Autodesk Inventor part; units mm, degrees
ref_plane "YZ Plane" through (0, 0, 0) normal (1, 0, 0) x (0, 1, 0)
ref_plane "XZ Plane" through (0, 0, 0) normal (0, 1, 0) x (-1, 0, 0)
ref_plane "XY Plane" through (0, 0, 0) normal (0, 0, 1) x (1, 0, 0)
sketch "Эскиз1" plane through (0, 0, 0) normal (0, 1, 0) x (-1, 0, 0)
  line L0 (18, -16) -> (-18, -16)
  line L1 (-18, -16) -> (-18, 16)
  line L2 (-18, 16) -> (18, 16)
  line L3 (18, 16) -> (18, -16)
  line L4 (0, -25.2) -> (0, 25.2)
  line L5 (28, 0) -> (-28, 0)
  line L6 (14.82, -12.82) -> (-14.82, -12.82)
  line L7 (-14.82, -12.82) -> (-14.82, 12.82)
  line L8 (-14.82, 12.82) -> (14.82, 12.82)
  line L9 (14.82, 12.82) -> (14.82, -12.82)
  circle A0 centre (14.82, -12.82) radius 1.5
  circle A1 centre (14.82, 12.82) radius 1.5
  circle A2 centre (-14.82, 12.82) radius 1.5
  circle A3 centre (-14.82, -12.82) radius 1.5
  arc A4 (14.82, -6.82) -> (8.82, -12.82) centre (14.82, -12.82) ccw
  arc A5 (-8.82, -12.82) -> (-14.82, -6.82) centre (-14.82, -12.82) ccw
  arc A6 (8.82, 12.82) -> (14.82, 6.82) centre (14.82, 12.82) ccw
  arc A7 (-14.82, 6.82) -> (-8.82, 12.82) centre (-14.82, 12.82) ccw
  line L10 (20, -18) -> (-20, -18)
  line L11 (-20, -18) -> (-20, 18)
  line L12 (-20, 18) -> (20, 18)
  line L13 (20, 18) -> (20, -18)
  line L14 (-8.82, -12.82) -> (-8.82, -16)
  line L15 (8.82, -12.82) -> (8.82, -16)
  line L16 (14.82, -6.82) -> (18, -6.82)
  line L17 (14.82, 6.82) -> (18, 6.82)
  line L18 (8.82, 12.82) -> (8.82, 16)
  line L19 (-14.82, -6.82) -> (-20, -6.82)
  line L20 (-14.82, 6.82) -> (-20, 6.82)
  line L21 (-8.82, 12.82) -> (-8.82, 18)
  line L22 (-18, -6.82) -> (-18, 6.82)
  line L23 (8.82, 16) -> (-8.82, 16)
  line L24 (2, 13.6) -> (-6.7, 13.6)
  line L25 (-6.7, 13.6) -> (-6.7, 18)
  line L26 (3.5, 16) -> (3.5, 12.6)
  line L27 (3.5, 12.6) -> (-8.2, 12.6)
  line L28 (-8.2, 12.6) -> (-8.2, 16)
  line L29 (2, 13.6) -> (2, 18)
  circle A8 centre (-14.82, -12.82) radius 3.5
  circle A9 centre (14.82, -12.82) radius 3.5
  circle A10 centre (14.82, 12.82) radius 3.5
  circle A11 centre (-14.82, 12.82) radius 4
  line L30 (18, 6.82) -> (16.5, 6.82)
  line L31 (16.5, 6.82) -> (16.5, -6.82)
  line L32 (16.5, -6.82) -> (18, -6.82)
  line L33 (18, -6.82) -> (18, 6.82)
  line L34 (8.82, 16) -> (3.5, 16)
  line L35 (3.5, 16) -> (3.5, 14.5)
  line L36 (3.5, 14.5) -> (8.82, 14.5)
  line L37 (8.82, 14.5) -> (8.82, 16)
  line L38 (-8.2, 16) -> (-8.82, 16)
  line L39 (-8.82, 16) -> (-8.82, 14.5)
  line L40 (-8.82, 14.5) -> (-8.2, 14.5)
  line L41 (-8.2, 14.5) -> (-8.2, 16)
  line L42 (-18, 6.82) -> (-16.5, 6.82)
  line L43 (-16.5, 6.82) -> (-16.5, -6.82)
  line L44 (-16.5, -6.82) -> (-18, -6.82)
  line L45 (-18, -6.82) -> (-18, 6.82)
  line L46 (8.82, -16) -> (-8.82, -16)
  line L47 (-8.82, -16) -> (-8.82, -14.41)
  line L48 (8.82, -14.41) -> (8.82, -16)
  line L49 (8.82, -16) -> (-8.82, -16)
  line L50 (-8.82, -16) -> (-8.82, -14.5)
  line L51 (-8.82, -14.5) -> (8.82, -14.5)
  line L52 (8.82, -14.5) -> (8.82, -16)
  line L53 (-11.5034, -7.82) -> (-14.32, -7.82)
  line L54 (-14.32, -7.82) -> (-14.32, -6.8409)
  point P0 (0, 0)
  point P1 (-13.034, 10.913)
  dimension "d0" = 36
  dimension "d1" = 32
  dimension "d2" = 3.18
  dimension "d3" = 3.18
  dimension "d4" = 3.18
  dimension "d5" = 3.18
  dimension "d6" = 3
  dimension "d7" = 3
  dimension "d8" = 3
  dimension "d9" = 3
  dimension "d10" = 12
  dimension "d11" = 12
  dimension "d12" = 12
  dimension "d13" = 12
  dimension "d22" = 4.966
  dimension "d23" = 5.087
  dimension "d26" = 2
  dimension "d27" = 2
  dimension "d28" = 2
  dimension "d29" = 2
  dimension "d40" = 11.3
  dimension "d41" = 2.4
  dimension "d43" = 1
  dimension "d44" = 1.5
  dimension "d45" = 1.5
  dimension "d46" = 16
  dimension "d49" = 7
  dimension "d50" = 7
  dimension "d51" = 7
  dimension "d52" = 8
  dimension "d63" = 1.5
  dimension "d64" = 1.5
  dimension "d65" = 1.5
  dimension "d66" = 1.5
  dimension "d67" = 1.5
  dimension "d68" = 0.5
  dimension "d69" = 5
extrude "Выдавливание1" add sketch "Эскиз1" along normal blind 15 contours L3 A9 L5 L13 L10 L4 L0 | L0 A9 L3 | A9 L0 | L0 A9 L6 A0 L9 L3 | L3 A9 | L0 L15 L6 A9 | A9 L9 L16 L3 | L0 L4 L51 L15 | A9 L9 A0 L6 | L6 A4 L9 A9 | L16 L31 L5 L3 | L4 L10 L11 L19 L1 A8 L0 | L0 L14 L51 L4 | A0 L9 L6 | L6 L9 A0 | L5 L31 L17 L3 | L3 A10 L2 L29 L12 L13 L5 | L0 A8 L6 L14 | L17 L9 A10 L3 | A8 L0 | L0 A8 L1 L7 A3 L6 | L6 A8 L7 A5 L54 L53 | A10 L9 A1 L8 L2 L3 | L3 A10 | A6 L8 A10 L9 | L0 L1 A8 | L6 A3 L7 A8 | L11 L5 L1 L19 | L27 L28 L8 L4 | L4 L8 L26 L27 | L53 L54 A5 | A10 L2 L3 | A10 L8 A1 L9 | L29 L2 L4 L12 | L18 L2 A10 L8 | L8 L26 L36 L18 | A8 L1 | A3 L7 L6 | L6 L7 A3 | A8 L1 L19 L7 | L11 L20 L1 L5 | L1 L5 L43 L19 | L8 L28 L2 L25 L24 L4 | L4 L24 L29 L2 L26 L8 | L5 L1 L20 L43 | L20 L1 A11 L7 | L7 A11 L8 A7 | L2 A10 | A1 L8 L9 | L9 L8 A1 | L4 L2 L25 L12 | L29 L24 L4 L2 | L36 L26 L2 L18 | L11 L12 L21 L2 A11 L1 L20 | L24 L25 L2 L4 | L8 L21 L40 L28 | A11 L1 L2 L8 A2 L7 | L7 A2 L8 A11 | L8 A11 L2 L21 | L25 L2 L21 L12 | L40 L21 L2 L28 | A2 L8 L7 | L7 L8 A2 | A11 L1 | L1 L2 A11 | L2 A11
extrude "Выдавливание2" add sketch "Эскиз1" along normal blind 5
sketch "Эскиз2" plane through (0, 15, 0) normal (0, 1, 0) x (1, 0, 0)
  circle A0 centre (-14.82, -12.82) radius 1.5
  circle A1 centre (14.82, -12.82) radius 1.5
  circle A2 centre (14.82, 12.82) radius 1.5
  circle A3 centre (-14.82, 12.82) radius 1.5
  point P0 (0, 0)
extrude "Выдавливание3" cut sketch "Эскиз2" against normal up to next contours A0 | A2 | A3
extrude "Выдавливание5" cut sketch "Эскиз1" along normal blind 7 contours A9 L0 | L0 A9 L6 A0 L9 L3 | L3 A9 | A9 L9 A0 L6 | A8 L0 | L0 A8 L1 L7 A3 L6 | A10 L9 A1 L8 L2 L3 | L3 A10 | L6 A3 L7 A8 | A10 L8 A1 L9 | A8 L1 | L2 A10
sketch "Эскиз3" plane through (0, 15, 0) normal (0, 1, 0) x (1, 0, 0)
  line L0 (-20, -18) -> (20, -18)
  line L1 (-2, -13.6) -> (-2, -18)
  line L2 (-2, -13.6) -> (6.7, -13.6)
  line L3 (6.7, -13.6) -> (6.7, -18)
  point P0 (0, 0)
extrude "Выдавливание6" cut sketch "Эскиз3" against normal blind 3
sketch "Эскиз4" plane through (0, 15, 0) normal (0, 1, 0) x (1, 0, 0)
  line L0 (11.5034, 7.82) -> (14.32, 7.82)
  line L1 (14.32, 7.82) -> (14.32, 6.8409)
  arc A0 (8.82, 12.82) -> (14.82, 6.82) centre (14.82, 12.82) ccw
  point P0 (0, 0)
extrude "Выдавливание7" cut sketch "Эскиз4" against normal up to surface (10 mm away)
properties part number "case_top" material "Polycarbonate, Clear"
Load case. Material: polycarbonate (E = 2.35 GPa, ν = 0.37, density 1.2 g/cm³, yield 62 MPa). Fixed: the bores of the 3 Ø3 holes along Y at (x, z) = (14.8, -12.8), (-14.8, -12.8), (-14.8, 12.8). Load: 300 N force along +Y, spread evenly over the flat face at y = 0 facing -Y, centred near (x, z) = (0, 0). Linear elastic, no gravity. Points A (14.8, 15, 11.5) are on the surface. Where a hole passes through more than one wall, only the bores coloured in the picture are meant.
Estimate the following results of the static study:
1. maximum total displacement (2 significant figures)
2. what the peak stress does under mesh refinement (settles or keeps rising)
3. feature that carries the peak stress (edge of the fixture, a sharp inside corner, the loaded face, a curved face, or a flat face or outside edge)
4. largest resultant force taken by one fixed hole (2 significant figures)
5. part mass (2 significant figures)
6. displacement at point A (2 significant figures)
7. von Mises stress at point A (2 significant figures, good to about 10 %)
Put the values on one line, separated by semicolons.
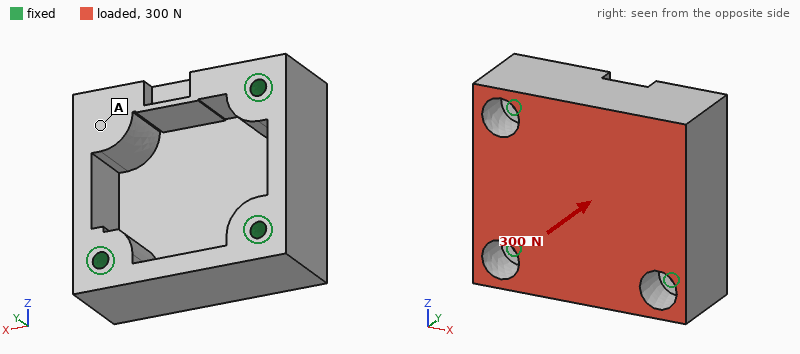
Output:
95 µm; keeps rising; edge of the fixture; 150 N; 16 g; 71 µm; 0.81 MPa
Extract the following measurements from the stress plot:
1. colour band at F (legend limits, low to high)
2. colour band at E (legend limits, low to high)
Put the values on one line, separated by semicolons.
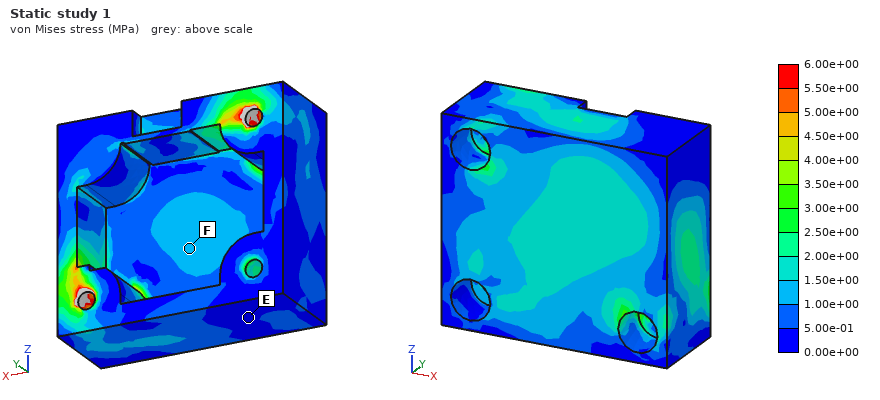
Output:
1.00e+00 to 1.50e+00 MPa; 0.00e+00 to 5.00e-01 MPa
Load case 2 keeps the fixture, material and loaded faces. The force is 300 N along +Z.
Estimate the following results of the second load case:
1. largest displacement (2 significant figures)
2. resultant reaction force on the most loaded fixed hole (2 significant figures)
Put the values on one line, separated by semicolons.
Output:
74 µm; 140 N
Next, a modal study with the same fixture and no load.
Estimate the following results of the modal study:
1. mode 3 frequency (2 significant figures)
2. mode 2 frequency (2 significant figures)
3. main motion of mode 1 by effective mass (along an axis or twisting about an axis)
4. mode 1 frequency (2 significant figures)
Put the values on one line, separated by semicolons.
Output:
6200 Hz; 5200 Hz; along Y; 2700 Hz
